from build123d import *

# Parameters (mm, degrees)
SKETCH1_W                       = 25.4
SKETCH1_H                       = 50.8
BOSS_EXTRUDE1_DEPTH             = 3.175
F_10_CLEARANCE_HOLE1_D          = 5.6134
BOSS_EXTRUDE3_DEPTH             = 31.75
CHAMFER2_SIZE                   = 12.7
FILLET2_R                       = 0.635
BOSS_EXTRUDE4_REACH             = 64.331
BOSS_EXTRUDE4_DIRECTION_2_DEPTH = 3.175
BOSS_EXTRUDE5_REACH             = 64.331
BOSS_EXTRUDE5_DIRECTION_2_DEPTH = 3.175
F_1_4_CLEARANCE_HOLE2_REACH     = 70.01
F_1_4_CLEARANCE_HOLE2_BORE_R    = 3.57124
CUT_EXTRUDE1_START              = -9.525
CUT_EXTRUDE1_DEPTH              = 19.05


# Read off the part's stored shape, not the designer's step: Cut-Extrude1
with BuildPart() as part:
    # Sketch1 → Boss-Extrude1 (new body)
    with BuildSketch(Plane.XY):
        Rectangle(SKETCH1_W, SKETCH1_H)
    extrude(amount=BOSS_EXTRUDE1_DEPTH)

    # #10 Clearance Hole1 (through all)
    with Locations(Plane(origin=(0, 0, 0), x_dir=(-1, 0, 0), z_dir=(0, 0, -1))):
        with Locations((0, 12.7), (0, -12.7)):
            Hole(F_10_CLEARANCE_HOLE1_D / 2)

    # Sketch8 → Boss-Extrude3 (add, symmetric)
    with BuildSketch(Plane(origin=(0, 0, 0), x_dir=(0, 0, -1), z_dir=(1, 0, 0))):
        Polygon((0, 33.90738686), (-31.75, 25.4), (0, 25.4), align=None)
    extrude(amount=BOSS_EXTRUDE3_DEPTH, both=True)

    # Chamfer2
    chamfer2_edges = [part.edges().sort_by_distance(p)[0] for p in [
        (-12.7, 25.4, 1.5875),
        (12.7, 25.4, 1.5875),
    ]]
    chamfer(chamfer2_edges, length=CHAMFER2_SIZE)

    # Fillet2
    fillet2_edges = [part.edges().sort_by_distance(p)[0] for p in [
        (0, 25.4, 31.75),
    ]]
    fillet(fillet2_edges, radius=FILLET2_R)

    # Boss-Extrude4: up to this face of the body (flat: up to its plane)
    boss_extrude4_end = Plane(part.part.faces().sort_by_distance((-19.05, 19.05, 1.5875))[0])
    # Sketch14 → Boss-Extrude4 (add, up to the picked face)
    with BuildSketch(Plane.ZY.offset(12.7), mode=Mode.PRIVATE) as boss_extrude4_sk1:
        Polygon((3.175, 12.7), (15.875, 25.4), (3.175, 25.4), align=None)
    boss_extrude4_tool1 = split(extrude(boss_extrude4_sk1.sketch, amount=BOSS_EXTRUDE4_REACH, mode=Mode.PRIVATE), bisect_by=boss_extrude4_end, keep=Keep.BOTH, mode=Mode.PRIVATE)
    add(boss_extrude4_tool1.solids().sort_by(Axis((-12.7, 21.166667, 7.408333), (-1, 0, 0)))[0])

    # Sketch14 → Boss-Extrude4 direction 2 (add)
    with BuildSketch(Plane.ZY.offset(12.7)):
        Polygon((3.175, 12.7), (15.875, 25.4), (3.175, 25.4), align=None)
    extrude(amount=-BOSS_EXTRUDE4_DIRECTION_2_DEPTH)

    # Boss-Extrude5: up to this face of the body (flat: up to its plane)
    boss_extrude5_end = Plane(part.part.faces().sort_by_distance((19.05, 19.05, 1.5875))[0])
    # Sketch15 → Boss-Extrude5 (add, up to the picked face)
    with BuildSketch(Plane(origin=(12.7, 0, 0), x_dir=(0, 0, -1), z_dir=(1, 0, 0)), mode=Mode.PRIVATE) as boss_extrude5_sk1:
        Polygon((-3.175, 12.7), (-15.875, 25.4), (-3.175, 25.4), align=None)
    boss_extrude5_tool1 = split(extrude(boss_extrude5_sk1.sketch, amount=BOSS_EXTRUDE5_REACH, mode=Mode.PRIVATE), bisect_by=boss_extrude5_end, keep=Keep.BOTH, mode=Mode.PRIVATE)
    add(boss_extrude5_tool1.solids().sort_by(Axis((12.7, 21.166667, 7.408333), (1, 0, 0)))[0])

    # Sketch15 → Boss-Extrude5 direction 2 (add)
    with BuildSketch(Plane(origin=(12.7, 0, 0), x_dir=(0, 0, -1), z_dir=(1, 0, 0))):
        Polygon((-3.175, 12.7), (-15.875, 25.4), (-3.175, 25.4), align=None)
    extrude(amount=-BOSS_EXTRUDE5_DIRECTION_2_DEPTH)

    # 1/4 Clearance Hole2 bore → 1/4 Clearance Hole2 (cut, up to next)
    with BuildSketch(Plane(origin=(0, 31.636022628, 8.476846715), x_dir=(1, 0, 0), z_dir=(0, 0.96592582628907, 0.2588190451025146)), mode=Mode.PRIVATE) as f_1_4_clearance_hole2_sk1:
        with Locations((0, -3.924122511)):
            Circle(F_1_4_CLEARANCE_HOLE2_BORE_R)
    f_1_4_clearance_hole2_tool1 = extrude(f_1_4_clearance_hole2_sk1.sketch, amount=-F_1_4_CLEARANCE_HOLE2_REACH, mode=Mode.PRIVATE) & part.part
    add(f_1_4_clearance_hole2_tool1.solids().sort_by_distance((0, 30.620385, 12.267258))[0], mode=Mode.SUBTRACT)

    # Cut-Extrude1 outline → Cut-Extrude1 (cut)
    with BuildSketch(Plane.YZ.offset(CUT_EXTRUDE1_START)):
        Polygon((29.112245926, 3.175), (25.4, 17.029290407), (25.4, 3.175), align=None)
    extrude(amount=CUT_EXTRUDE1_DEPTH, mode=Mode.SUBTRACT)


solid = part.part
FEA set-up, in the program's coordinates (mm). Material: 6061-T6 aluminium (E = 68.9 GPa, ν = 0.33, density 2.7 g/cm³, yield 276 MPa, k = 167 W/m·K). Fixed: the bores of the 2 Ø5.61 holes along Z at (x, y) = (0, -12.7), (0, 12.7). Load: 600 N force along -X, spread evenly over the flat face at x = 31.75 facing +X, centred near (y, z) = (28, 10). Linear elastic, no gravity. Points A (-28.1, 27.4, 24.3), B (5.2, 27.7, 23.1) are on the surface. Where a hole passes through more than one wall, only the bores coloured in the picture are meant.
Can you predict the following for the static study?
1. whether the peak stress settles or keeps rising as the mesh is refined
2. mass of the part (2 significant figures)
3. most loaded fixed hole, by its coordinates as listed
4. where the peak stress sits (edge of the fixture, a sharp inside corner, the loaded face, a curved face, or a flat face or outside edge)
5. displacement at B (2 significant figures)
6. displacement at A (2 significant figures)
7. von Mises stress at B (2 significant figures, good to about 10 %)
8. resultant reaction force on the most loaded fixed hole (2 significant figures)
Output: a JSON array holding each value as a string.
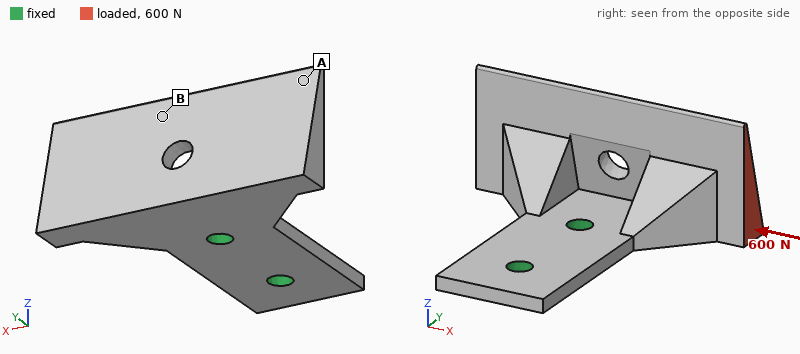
["keeps rising", "38 g", "(0, 12.7)", "edge of the fixture", "0.10 mm", "0.16 mm", "19 MPa", "840 N"]
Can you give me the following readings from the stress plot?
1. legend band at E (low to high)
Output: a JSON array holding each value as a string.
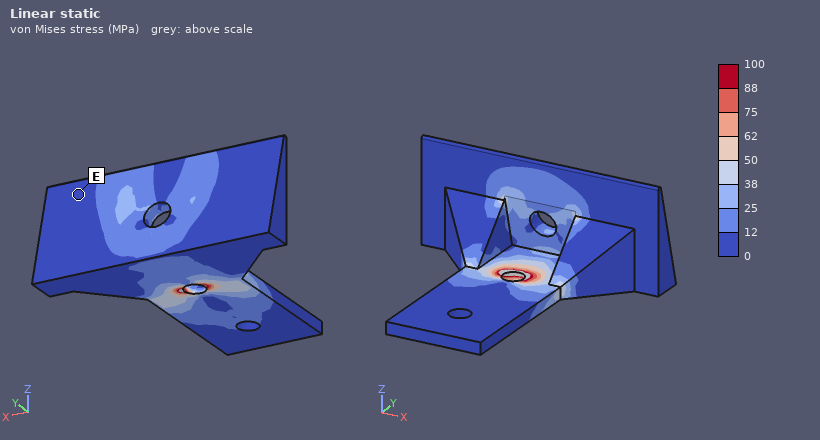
["0 to 12 MPa"]
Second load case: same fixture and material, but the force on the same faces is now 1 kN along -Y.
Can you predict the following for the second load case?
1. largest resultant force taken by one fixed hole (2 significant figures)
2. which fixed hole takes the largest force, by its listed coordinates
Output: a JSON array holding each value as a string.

["1.1 kN", "(0, 12.7)"]
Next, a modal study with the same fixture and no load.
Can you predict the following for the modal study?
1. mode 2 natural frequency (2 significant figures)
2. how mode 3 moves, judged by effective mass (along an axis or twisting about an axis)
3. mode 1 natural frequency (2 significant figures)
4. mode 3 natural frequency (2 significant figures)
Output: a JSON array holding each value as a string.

["2000 Hz", "along X", "1600 Hz", "5000 Hz"]
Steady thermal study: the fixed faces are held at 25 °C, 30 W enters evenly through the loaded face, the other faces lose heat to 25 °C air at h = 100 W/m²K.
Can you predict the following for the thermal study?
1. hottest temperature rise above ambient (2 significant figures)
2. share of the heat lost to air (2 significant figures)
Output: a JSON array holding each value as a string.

["45 K", "33 %"]
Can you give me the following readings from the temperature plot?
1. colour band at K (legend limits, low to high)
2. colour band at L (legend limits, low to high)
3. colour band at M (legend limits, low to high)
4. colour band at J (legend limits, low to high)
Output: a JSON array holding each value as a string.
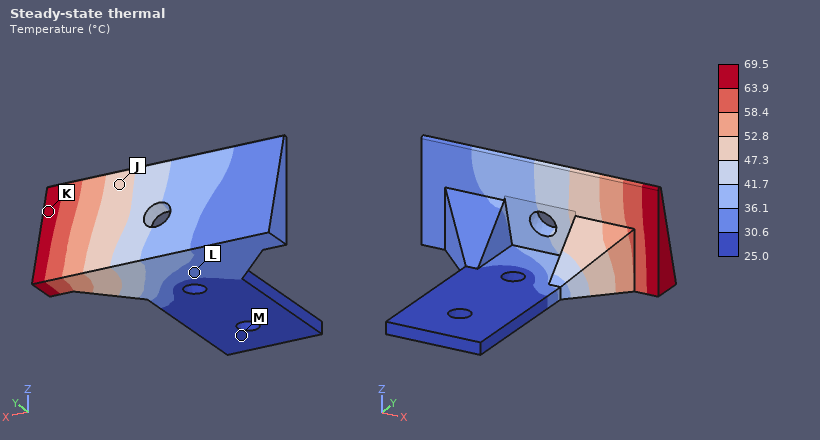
["63.9 to 69.5 °C", "30.6 to 36.1 °C", "25.0 to 30.6 °C", "47.3 to 52.8 °C"]
